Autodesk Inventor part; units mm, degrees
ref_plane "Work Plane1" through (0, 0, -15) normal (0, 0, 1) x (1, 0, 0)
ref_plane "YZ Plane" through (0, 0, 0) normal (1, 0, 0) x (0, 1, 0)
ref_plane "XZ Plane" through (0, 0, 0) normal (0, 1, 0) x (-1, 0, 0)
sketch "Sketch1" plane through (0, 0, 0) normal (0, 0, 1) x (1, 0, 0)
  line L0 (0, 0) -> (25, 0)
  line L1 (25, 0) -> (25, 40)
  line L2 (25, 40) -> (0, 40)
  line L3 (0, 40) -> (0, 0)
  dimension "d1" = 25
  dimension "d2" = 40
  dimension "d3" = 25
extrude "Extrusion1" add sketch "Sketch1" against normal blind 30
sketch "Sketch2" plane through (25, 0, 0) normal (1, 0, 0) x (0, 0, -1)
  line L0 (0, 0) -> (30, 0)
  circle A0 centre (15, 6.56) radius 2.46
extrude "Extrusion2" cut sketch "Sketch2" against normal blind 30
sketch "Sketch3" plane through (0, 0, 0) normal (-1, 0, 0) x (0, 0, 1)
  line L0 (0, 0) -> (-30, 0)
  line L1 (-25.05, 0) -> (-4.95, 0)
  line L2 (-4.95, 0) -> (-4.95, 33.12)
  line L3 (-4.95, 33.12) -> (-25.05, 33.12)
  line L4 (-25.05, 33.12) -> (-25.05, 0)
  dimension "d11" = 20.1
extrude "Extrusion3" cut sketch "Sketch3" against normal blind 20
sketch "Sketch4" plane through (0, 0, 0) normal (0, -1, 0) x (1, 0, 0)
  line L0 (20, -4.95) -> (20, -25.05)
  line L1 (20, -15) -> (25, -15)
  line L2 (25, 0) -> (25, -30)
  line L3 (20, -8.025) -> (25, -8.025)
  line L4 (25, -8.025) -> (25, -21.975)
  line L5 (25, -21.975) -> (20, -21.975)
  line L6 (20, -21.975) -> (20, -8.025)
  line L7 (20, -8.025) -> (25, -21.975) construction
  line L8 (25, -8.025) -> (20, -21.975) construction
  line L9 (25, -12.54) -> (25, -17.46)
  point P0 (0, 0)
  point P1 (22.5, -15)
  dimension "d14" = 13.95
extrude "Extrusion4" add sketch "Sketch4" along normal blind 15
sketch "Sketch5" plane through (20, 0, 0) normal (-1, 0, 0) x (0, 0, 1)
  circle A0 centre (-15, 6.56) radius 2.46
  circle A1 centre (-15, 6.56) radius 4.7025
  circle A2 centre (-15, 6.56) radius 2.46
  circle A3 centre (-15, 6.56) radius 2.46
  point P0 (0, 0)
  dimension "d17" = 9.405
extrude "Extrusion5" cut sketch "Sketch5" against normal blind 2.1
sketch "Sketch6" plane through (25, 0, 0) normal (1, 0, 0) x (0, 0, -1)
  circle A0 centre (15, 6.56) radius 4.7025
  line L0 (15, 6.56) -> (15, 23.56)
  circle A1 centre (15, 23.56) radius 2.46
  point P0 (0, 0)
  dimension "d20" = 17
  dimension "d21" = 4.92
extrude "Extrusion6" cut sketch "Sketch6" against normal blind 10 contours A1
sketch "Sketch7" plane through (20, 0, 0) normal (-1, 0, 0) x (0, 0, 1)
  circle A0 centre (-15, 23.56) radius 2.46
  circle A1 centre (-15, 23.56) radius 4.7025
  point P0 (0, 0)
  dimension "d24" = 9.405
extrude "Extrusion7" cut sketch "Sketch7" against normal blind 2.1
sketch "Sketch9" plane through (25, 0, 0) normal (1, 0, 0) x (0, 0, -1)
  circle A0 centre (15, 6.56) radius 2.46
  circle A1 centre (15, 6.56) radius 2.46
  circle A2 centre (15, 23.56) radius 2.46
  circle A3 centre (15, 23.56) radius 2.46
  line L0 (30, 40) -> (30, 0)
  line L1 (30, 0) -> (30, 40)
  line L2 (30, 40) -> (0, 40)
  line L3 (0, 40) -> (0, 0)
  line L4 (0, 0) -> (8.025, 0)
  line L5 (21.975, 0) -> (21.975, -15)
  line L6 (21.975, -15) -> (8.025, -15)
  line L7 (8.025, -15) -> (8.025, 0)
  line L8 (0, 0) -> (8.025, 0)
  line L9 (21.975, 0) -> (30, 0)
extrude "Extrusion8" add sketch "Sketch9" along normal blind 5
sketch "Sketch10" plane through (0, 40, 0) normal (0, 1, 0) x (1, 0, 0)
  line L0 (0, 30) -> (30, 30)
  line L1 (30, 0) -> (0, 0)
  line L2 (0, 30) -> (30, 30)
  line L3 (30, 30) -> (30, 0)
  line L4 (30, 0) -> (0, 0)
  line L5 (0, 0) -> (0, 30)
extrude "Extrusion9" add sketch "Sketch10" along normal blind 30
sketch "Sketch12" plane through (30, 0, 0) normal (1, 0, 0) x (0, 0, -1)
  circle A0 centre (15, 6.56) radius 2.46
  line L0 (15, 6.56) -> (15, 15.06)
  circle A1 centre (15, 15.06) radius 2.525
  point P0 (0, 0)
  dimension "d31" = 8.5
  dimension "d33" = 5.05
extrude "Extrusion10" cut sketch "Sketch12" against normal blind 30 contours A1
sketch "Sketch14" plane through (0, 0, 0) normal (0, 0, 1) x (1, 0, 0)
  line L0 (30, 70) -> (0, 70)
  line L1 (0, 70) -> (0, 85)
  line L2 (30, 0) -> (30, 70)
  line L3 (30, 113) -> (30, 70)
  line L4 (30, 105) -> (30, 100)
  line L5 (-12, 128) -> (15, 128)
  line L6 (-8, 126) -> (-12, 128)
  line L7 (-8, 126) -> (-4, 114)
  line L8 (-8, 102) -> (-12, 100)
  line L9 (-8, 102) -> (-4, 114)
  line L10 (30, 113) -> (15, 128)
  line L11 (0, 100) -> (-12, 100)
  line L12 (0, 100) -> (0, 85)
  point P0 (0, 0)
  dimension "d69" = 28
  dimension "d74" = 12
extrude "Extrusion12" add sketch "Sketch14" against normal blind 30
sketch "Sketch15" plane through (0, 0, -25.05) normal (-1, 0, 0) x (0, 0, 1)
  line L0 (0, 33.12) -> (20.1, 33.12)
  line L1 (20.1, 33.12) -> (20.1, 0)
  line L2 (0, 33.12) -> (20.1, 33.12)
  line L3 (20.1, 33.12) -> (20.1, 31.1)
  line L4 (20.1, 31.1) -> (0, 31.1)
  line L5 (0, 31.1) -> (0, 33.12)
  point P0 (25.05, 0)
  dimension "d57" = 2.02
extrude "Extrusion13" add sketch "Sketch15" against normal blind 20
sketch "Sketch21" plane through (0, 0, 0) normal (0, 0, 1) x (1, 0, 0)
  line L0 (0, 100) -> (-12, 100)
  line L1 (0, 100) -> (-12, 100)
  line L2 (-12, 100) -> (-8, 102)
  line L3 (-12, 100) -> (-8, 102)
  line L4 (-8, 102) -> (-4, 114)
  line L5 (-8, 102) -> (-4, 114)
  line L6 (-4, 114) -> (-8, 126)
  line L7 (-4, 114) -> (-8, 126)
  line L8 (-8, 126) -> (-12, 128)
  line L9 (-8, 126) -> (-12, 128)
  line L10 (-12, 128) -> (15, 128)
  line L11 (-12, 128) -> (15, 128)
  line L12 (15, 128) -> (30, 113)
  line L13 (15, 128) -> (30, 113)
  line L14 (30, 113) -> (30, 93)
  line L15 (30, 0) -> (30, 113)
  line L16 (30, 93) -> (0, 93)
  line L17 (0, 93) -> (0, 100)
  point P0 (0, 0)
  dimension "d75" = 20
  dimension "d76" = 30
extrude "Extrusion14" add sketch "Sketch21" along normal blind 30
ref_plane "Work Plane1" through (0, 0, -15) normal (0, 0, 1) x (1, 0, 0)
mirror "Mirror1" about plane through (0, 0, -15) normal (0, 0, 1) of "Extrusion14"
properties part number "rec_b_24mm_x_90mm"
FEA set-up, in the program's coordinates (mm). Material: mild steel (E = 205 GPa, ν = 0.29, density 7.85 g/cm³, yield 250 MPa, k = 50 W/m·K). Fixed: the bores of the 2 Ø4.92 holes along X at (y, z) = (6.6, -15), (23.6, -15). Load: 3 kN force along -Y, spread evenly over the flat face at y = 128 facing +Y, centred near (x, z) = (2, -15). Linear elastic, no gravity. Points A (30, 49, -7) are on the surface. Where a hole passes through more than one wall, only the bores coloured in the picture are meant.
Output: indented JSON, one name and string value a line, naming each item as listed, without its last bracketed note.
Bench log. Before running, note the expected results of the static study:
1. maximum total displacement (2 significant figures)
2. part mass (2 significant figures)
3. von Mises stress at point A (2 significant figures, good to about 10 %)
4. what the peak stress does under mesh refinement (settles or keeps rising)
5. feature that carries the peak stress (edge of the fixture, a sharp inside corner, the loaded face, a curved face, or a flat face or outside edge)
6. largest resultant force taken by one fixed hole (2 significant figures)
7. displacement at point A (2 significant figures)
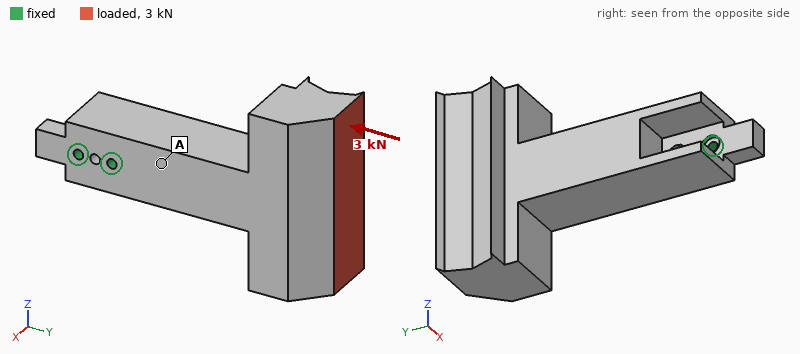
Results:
{
  "maximum total displacement": "74 µm",
  "part mass": "1.4 kg",
  "von Mises stress at point A": "5.4 MPa",
  "what the peak stress does under mesh refinement": "keeps rising",
  "feature that carries the peak stress": "edge of the fixture",
  "largest resultant force taken by one fixed hole": "3.4 kN",
  "displacement at point A": "14 µm"
}
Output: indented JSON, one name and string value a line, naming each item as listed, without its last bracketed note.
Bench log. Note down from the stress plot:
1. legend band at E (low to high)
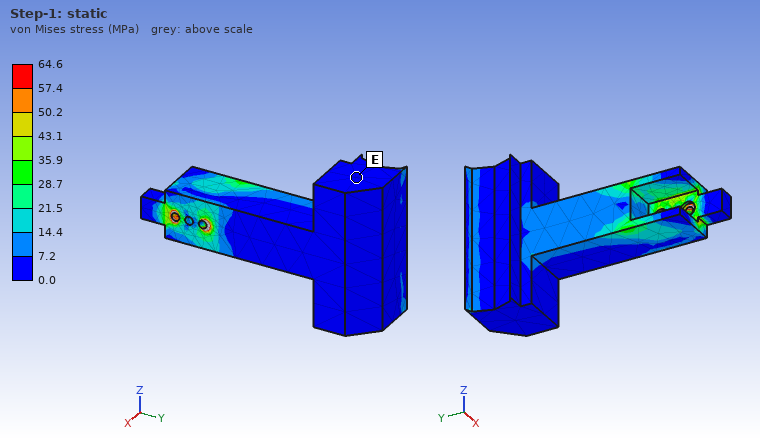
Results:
{
  "legend band at E": "0.0 to 7.2 MPa"
}
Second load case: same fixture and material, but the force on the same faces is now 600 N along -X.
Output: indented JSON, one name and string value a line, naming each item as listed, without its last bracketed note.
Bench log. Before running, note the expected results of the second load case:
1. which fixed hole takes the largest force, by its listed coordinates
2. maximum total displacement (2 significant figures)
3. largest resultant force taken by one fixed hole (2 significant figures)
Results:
{
  "which fixed hole takes the largest force, by its listed coordinates": "(23.6, -15)",
  "maximum total displacement": "67 µm",
  "largest resultant force taken by one fixed hole": "3.1 kN"
}
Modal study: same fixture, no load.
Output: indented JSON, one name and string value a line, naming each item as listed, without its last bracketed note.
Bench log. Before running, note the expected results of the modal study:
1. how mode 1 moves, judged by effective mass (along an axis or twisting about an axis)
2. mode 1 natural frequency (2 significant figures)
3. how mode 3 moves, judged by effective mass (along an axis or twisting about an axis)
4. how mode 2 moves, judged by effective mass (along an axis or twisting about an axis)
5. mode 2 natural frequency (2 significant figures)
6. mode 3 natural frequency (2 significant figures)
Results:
{
  "how mode 1 moves, judged by effective mass": "along X",
  "mode 1 natural frequency": "630 Hz",
  "how mode 3 moves, judged by effective mass": "twisting about Y",
  "how mode 2 moves, judged by effective mass": "along Z",
  "mode 2 natural frequency": "710 Hz",
  "mode 3 natural frequency": "1300 Hz"
}
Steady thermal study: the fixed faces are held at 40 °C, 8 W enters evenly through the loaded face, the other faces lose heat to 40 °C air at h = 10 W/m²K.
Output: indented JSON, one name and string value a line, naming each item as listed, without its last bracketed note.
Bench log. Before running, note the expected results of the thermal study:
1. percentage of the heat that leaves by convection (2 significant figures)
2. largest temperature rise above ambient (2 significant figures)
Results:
{
  "percentage of the heat that leaves by convection": "32 %",
  "largest temperature rise above ambient": "17 K"
}
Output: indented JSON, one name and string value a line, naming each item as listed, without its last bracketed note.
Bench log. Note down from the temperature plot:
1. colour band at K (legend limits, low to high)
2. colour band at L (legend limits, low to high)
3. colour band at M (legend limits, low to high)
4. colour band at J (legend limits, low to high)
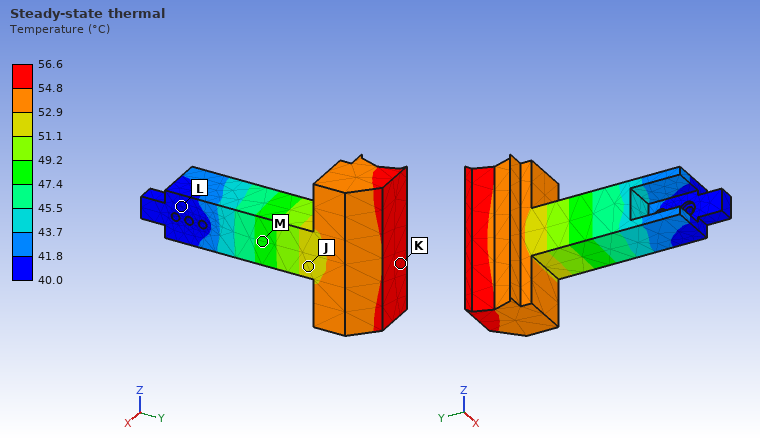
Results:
{
  "colour band at K": "54.8 to 56.6 °C",
  "colour band at L": "40.0 to 41.8 °C",
  "colour band at M": "47.4 to 49.2 °C",
  "colour band at J": "51.1 to 52.9 °C"
}
